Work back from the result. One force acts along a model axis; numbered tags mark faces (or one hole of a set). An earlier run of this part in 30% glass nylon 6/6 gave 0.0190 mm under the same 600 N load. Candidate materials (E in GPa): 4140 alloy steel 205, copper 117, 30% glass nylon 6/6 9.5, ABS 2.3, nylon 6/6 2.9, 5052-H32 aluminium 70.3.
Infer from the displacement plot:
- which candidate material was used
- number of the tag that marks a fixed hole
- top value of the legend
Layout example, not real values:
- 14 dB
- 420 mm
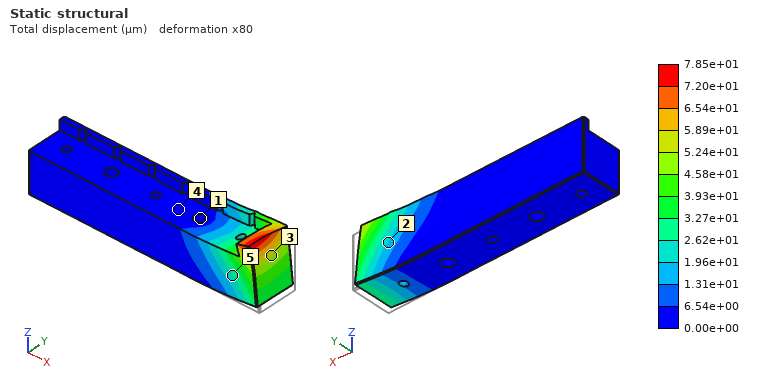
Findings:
- ABS
- 1
- 7.85e+01 µm
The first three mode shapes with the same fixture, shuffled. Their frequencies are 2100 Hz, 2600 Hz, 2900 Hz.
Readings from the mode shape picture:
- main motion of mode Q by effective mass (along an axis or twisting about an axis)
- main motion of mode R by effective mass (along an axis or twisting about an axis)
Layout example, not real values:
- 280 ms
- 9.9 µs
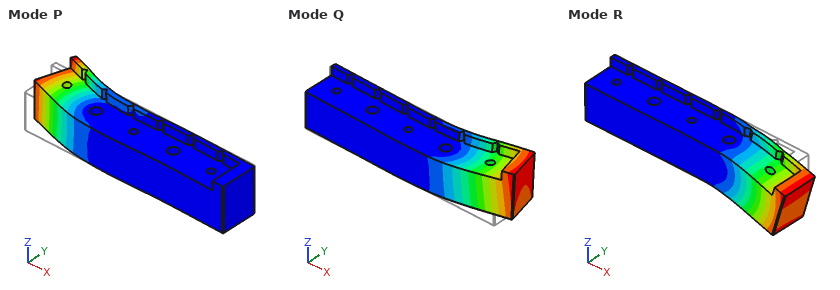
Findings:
- along Y
- along Z
